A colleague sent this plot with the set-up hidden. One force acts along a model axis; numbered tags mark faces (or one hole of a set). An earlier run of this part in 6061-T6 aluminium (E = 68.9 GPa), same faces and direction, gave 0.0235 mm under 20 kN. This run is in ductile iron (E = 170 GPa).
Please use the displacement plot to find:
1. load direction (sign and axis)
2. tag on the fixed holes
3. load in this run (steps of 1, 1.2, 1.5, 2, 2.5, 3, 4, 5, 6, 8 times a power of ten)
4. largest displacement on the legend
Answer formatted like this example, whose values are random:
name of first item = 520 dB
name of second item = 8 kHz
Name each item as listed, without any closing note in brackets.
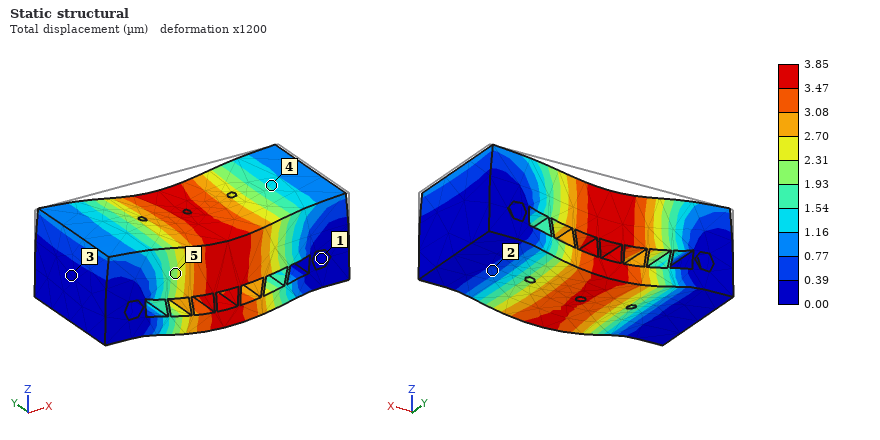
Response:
load direction = -Z
tag on the fixed holes = 1
load in this run = 8 kN
largest displacement on the legend = 3.85 µm
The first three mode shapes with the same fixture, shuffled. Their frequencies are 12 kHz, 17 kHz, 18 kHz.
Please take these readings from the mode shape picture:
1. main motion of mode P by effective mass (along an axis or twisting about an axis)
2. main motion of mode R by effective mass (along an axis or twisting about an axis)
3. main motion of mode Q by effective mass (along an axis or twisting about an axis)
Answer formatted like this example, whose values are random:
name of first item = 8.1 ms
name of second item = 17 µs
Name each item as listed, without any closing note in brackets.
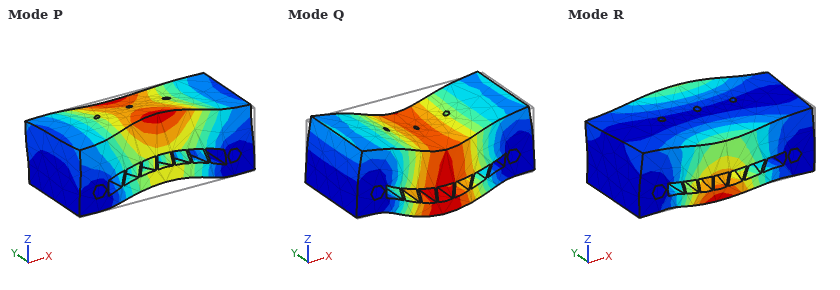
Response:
main motion of mode P by effective mass = along Y
main motion of mode R by effective mass = along Y
main motion of mode Q by effective mass = along Z
